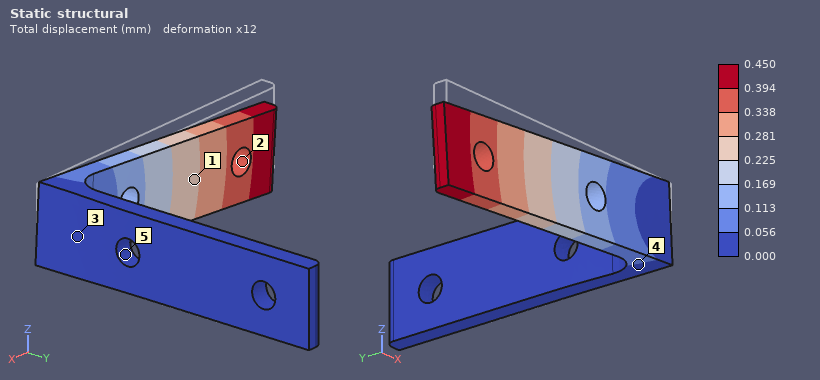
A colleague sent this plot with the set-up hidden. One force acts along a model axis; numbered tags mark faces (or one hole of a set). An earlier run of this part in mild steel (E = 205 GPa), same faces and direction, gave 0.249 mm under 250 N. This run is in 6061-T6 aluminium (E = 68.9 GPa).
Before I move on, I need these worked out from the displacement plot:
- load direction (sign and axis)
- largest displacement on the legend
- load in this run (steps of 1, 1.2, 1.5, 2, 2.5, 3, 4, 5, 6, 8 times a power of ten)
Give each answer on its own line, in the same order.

-Z
0.450 mm
150 N
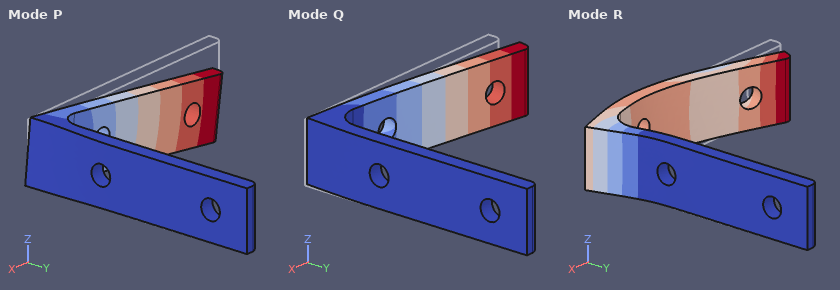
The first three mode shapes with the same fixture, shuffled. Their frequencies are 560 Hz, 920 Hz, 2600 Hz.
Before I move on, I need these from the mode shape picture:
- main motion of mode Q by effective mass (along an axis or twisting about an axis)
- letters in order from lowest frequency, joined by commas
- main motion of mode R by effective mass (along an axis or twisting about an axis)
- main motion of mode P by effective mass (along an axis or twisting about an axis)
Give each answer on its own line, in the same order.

along Y
Q, P, R
along X
along Z
